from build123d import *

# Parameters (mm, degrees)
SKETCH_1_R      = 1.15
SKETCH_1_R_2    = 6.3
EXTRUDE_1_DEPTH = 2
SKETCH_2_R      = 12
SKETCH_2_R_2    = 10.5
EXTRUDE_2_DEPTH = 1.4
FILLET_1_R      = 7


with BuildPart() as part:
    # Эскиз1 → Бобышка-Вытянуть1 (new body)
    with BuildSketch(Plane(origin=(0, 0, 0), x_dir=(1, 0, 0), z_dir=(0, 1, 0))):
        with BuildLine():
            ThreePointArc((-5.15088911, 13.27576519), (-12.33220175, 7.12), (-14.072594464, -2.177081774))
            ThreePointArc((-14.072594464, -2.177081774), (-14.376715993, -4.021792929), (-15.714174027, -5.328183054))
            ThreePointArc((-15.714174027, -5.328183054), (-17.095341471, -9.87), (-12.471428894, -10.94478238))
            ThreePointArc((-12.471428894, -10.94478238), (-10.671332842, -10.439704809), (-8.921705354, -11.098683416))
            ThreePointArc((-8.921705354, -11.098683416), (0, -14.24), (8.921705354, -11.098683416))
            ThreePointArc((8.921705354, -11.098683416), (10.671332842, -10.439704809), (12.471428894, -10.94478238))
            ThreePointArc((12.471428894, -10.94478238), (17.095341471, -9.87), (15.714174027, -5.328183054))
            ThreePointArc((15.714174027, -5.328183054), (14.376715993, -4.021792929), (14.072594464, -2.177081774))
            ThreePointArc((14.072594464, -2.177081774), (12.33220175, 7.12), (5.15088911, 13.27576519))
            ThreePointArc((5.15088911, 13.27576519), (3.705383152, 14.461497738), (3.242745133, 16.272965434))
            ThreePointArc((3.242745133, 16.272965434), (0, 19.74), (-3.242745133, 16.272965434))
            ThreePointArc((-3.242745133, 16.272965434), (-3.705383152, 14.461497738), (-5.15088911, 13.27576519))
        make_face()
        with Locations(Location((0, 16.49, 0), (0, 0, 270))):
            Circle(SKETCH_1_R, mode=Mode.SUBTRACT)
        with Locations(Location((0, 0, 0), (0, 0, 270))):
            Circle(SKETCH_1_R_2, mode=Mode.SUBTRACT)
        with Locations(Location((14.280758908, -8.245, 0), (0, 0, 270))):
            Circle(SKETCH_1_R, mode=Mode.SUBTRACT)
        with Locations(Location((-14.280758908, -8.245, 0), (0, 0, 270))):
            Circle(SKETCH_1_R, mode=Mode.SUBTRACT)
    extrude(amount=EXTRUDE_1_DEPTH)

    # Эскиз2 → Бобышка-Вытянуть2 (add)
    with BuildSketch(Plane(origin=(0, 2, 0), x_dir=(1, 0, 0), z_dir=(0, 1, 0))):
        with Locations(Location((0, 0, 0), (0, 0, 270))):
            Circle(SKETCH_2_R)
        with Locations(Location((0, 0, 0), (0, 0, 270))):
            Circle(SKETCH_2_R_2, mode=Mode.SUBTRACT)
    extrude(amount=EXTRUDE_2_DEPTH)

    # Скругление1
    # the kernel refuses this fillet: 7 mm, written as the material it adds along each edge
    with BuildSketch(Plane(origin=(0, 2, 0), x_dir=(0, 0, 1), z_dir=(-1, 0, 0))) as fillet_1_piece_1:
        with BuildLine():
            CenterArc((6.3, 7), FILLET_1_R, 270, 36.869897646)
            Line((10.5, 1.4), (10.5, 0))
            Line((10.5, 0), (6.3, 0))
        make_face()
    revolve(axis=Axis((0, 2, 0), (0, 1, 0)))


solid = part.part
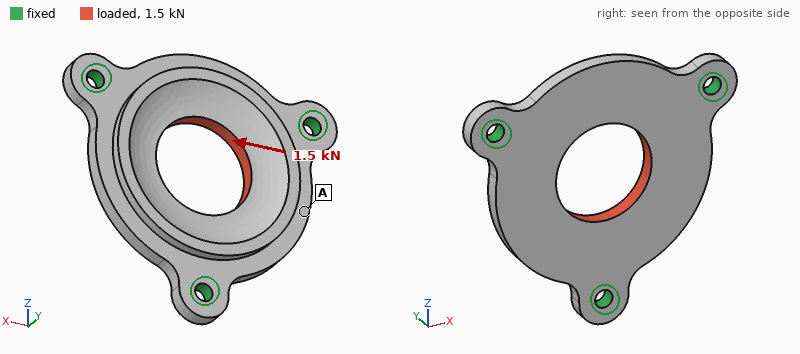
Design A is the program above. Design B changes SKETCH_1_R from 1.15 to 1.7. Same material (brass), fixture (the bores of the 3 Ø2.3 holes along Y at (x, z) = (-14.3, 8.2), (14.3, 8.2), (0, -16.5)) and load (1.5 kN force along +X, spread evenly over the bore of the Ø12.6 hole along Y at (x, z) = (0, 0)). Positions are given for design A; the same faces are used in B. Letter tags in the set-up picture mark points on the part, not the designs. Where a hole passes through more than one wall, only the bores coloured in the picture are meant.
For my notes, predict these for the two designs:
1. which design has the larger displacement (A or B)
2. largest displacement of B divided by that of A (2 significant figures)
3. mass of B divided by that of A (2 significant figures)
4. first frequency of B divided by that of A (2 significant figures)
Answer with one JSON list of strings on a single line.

["A", "0.87", "0.98", "1.1"]
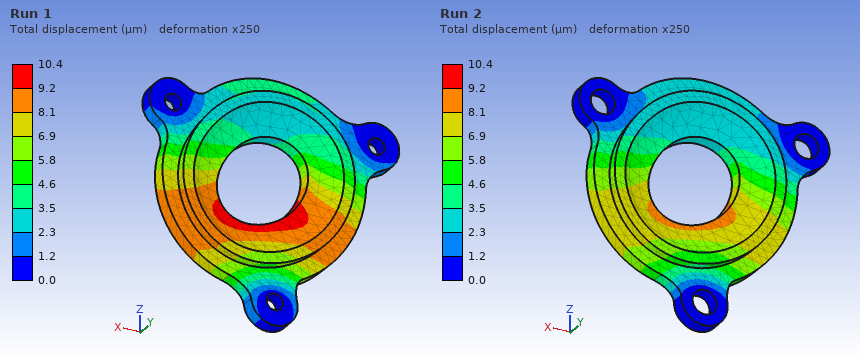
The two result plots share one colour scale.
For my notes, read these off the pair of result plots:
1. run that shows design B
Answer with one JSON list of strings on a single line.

["Run 2"]
